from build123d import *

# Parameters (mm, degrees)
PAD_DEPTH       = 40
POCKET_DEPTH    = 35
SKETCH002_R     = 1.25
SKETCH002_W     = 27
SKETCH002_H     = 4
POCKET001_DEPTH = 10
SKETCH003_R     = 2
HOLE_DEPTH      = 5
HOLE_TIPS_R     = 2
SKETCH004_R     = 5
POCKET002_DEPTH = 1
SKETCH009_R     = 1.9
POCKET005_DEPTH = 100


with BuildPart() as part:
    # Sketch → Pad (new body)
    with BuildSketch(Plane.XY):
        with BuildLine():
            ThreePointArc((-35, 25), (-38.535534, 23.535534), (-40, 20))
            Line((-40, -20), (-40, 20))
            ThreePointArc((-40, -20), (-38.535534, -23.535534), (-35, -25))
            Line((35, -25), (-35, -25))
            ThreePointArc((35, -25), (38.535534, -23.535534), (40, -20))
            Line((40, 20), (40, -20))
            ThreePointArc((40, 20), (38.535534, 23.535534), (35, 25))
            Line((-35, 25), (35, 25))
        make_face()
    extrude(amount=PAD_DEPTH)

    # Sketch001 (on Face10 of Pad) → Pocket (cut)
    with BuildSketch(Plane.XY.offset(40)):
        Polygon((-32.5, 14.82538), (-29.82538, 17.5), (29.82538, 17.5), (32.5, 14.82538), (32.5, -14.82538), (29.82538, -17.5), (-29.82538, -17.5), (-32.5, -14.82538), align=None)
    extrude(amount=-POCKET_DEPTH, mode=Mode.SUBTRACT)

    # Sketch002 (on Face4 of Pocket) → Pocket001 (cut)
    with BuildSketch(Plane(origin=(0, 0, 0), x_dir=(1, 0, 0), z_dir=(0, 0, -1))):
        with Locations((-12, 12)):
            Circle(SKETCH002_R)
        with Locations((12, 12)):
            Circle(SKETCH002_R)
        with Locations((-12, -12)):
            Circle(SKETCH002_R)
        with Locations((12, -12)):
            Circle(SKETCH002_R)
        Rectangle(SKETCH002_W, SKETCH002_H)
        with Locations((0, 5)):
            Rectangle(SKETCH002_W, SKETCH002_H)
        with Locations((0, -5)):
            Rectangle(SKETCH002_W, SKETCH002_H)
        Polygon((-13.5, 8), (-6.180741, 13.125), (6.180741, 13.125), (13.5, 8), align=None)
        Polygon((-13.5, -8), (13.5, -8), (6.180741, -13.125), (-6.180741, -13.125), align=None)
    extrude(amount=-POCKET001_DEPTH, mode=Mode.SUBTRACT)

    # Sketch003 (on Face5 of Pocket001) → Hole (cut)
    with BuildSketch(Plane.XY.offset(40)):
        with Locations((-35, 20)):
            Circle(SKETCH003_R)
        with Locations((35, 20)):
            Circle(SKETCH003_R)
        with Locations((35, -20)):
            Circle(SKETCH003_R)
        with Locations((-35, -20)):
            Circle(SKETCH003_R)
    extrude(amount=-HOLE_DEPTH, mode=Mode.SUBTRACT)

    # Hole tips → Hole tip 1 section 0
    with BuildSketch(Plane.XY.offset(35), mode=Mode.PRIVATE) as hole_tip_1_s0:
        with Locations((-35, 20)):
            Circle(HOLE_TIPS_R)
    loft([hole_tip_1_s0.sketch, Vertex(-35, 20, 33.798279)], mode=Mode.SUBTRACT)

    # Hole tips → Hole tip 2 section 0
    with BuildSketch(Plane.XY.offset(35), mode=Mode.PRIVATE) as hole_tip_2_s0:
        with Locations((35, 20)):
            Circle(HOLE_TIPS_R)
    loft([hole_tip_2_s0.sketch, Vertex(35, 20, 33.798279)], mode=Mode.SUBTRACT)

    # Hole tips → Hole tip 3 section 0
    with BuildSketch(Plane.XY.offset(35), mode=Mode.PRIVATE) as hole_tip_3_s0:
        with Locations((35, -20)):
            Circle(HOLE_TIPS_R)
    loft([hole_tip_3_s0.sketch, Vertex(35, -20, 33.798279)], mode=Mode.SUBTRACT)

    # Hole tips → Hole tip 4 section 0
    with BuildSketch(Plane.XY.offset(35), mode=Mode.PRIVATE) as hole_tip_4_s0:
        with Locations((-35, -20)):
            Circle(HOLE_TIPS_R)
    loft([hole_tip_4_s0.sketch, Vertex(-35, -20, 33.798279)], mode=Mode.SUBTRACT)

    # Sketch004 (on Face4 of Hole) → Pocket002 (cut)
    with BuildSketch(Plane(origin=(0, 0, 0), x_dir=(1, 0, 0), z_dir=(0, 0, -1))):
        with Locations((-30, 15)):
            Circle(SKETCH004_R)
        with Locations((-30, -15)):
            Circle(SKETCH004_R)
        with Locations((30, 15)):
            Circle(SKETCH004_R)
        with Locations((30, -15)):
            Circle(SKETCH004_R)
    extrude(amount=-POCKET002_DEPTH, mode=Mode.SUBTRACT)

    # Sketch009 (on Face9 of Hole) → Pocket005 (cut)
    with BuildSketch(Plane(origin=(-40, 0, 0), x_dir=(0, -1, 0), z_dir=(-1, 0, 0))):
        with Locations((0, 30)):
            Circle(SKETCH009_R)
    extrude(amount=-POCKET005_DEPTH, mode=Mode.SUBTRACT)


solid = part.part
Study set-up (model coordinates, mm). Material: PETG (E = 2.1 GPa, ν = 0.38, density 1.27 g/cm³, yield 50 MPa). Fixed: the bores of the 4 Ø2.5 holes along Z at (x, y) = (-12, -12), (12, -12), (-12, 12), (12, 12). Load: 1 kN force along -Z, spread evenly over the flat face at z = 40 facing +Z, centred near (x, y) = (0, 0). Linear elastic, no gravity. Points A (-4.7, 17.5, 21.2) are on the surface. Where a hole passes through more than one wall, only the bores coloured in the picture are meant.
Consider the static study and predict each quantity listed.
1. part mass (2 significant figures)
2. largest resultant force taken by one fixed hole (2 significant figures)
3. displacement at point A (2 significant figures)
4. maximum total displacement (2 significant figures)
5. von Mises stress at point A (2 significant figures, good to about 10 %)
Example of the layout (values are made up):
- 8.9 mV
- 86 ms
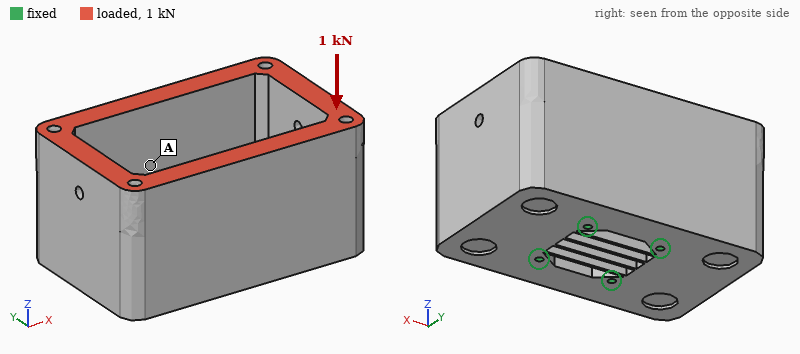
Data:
- 97 g
- 260 N
- 0.11 mm
- 0.13 mm
- 2.0 MPa
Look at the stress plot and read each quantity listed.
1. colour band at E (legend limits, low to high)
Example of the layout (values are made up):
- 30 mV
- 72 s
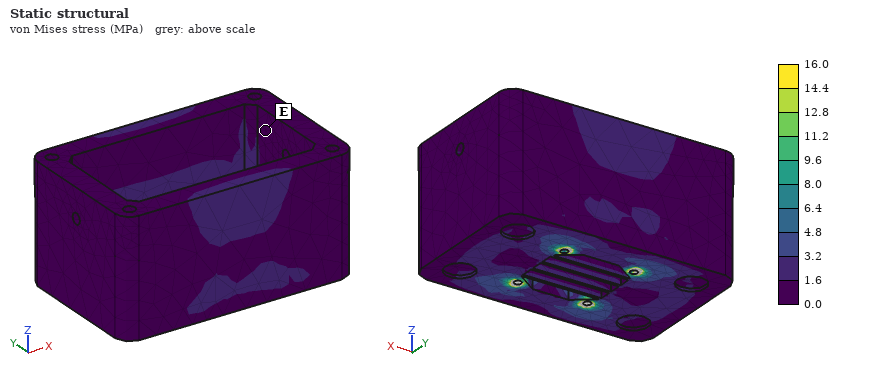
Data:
- 0.0 to 1.6 MPa
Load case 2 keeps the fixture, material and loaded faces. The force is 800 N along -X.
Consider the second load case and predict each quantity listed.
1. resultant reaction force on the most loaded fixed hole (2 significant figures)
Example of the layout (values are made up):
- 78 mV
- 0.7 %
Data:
- 570 N
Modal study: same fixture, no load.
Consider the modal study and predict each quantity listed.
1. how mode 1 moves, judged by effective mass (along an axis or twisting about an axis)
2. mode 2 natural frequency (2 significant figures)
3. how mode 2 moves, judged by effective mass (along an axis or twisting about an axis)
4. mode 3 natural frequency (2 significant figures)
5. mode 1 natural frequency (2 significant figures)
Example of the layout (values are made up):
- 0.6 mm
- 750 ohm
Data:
- along X
- 720 Hz
- along Y
- 1000 Hz
- 680 Hz
